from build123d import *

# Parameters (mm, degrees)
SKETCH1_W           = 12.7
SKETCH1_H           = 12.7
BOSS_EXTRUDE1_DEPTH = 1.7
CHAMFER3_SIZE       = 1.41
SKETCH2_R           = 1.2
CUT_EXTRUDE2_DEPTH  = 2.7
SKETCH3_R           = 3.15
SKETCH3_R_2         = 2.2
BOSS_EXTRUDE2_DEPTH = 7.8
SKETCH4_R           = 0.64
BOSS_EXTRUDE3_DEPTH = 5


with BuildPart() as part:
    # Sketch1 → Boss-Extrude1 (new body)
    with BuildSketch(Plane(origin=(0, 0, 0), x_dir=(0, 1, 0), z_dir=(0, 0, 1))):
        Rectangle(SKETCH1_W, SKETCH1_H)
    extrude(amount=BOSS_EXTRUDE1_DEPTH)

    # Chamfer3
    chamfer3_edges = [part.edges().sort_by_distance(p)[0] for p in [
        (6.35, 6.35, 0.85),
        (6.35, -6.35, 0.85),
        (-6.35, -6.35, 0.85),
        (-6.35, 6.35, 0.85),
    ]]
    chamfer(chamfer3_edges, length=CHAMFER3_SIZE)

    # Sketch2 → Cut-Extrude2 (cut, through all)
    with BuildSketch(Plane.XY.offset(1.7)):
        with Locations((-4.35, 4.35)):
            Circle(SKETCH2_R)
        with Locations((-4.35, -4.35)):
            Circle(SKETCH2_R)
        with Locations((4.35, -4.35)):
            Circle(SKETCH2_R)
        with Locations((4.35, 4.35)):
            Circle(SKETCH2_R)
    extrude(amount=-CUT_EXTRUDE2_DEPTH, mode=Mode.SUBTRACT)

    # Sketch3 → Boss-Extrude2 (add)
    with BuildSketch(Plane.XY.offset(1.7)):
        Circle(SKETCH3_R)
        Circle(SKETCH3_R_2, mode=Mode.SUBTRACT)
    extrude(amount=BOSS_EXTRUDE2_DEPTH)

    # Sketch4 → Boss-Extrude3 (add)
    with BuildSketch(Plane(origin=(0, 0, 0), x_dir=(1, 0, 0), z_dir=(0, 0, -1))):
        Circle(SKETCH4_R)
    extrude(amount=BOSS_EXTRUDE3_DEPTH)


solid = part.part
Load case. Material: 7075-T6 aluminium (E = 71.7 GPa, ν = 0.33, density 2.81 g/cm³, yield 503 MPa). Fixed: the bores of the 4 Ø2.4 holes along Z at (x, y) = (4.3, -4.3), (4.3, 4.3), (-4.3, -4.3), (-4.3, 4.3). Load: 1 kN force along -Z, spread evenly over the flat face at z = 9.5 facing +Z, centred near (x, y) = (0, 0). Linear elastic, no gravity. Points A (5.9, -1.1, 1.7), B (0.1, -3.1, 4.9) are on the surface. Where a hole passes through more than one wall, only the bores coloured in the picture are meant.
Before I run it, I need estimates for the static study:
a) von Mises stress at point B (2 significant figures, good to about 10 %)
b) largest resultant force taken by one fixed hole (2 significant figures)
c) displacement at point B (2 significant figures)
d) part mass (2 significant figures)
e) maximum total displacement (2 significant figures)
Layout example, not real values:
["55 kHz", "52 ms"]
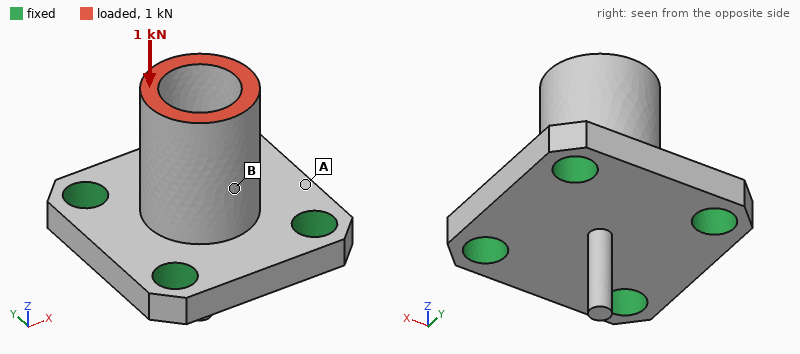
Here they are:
["56 MPa", "260 N", "10 µm", "1.0 g", "14 µm"]
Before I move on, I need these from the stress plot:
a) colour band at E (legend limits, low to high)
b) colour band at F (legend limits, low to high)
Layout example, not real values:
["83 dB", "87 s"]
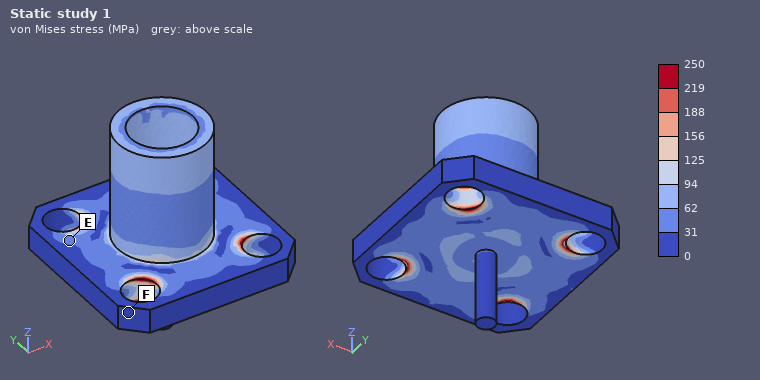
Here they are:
["31 to 62 MPa", "0 to 31 MPa"]
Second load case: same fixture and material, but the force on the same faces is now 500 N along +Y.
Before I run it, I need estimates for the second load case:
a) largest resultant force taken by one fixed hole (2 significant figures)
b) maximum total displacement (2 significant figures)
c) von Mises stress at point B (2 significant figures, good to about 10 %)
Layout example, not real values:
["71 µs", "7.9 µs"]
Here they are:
["340 N", "70 µm", "110 MPa"]
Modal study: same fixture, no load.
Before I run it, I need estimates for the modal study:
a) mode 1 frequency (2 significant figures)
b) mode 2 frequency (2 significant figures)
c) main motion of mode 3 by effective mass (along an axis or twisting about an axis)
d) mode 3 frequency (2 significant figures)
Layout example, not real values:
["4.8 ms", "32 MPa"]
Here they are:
["31 kHz", "31 kHz", "along X", "40 kHz"]
